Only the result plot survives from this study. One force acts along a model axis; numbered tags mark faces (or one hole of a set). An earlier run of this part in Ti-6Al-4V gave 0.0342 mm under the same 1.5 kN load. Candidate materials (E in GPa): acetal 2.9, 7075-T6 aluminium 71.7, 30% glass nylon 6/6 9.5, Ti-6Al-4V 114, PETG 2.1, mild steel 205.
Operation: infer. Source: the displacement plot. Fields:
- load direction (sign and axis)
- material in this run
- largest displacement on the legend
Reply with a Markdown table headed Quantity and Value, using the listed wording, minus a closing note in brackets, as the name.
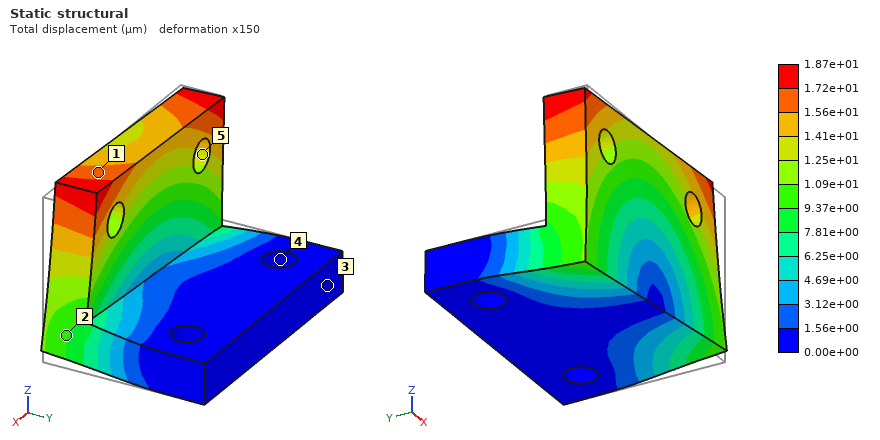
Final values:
| Quantity | Value |
|---|---|
| load direction | -X |
| material in this run | mild steel |
| largest displacement on the legend | 1.87e+01 µm |
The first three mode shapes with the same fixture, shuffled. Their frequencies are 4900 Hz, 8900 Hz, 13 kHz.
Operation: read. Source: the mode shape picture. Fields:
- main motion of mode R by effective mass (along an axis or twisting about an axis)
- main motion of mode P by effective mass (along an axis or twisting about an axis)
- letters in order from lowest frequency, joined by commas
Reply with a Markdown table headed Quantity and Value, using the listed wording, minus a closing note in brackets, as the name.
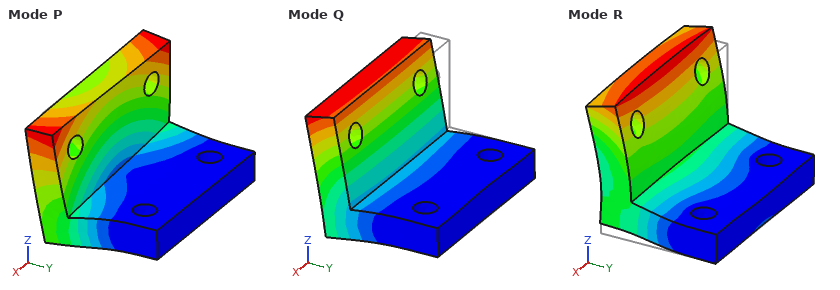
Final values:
| Quantity | Value |
|---|---|
| main motion of mode R by effective mass | along Z |
| main motion of mode P by effective mass | along X |
| letters in order from lowest frequency, joined by commas | Q, P, R |
